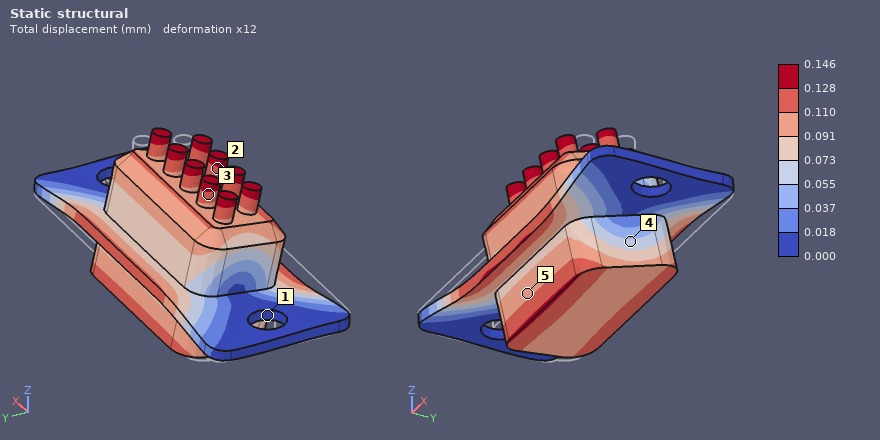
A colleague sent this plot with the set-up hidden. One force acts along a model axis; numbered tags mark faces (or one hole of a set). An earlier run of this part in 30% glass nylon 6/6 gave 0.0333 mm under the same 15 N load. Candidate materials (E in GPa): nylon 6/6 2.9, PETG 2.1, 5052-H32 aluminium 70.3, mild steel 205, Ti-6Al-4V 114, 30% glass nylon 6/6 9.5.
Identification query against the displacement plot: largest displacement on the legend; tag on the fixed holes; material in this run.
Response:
0.146 mm
1
PETG
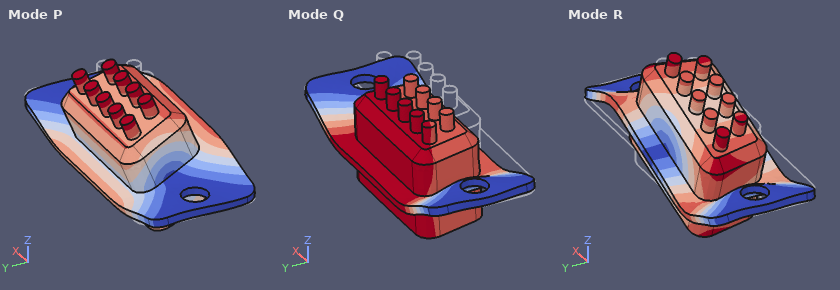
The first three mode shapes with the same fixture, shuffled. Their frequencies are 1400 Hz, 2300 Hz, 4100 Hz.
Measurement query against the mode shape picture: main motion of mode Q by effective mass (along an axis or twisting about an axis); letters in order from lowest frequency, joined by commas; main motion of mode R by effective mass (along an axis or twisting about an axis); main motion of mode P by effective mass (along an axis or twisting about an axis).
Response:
along Z
P, Q, R
twisting about Y
twisting about X
